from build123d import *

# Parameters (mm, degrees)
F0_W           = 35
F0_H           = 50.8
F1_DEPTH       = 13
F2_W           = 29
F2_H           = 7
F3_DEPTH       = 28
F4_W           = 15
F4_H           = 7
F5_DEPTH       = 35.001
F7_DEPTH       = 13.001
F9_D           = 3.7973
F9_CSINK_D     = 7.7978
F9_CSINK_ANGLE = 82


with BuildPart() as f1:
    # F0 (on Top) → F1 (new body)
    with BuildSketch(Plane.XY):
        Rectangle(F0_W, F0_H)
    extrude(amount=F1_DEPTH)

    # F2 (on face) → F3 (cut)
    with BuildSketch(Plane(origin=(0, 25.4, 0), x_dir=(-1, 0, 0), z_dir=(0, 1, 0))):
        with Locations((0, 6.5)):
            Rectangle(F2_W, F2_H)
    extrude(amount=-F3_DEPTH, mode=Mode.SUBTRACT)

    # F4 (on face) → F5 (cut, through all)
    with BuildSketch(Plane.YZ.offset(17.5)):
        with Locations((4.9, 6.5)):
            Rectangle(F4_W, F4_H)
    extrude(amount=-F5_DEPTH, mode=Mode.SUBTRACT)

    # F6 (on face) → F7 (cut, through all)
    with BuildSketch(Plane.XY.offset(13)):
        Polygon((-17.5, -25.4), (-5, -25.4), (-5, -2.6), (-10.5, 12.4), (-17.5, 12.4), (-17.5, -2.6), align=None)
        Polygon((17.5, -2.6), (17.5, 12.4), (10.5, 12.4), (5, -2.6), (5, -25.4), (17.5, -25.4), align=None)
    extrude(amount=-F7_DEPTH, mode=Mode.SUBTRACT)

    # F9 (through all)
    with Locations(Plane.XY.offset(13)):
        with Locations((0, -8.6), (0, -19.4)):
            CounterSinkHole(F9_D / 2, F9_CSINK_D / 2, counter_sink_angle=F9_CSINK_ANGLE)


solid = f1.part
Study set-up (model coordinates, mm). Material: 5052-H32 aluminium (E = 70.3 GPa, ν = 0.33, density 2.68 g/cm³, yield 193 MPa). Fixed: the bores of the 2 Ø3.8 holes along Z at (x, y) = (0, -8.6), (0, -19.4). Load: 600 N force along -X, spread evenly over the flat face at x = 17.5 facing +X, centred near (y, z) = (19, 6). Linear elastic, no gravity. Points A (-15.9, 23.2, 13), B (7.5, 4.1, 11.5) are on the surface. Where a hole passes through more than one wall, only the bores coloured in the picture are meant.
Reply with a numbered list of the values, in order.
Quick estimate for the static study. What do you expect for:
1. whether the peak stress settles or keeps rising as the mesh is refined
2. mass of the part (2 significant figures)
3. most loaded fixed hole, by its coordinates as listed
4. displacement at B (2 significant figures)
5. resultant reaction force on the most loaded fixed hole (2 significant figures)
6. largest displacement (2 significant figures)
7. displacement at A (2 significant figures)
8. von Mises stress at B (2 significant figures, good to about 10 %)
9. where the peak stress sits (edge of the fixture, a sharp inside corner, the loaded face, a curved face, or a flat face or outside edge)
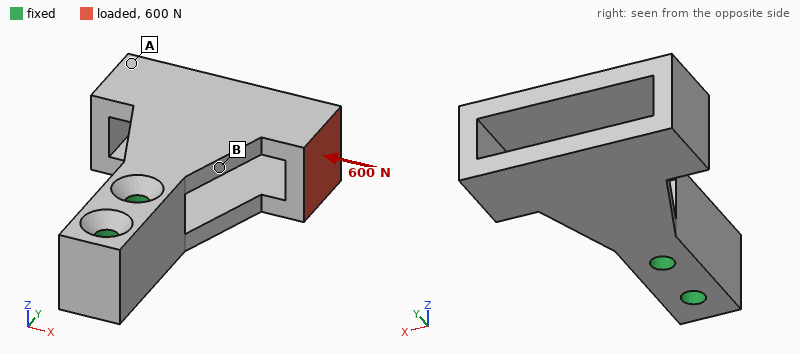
1. keeps rising
2. 19 g
3. (0, -8.6)
4. 0.044 mm
5. 1.2 kN
6. 0.15 mm
7. 0.13 mm
8. 31 MPa
9. edge of the fixture
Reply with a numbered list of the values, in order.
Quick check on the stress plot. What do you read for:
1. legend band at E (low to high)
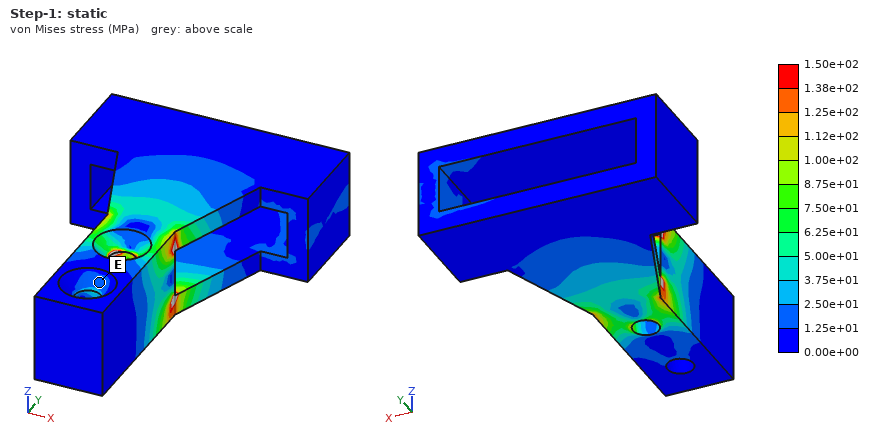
1. 1.25e+01 to 2.50e+01 MPa
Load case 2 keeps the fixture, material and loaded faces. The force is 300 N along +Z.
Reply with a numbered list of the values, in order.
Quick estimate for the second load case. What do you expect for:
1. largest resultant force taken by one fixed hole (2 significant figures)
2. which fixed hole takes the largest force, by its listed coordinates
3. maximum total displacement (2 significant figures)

1. 410 N
2. (0, -8.6)
3. 0.20 mm
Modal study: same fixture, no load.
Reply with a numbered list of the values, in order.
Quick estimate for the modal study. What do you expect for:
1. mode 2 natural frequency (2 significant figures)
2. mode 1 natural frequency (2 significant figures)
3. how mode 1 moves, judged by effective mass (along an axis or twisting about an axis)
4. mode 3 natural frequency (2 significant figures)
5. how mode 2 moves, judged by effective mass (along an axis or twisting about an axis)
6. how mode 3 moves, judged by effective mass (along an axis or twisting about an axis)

1. 3600 Hz
2. 2700 Hz
3. along Z
4. 4400 Hz
5. along X
6. twisting about Y
